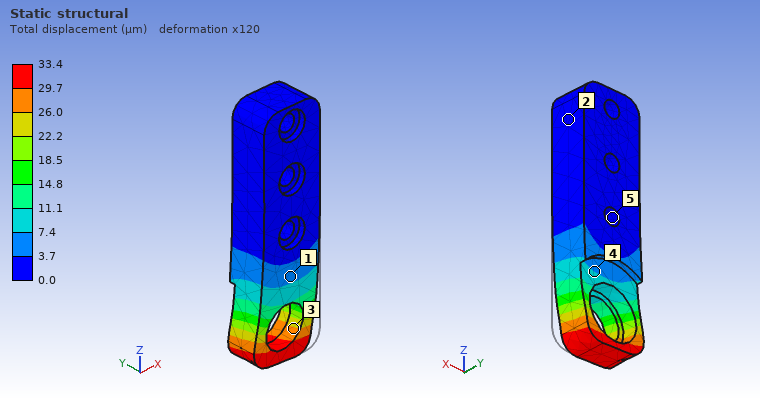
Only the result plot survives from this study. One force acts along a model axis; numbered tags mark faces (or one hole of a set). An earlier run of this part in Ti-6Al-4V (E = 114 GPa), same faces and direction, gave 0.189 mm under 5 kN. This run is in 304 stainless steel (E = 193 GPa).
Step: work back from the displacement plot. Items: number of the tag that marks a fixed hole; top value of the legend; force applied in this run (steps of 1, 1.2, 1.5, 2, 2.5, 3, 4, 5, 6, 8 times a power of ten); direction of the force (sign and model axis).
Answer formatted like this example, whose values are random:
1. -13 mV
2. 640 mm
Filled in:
1. 5
2. 33.4 µm
3. 1.5 kN
4. -X
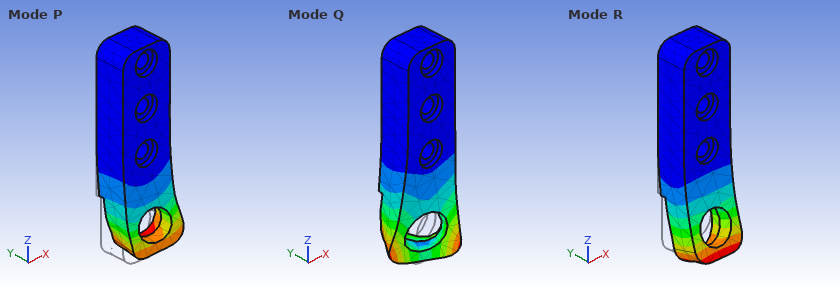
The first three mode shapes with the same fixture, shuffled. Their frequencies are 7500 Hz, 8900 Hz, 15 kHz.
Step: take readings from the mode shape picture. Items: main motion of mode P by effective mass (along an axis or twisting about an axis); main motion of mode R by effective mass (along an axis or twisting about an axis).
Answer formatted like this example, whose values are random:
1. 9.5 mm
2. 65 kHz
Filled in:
1. along X
2. along Y
